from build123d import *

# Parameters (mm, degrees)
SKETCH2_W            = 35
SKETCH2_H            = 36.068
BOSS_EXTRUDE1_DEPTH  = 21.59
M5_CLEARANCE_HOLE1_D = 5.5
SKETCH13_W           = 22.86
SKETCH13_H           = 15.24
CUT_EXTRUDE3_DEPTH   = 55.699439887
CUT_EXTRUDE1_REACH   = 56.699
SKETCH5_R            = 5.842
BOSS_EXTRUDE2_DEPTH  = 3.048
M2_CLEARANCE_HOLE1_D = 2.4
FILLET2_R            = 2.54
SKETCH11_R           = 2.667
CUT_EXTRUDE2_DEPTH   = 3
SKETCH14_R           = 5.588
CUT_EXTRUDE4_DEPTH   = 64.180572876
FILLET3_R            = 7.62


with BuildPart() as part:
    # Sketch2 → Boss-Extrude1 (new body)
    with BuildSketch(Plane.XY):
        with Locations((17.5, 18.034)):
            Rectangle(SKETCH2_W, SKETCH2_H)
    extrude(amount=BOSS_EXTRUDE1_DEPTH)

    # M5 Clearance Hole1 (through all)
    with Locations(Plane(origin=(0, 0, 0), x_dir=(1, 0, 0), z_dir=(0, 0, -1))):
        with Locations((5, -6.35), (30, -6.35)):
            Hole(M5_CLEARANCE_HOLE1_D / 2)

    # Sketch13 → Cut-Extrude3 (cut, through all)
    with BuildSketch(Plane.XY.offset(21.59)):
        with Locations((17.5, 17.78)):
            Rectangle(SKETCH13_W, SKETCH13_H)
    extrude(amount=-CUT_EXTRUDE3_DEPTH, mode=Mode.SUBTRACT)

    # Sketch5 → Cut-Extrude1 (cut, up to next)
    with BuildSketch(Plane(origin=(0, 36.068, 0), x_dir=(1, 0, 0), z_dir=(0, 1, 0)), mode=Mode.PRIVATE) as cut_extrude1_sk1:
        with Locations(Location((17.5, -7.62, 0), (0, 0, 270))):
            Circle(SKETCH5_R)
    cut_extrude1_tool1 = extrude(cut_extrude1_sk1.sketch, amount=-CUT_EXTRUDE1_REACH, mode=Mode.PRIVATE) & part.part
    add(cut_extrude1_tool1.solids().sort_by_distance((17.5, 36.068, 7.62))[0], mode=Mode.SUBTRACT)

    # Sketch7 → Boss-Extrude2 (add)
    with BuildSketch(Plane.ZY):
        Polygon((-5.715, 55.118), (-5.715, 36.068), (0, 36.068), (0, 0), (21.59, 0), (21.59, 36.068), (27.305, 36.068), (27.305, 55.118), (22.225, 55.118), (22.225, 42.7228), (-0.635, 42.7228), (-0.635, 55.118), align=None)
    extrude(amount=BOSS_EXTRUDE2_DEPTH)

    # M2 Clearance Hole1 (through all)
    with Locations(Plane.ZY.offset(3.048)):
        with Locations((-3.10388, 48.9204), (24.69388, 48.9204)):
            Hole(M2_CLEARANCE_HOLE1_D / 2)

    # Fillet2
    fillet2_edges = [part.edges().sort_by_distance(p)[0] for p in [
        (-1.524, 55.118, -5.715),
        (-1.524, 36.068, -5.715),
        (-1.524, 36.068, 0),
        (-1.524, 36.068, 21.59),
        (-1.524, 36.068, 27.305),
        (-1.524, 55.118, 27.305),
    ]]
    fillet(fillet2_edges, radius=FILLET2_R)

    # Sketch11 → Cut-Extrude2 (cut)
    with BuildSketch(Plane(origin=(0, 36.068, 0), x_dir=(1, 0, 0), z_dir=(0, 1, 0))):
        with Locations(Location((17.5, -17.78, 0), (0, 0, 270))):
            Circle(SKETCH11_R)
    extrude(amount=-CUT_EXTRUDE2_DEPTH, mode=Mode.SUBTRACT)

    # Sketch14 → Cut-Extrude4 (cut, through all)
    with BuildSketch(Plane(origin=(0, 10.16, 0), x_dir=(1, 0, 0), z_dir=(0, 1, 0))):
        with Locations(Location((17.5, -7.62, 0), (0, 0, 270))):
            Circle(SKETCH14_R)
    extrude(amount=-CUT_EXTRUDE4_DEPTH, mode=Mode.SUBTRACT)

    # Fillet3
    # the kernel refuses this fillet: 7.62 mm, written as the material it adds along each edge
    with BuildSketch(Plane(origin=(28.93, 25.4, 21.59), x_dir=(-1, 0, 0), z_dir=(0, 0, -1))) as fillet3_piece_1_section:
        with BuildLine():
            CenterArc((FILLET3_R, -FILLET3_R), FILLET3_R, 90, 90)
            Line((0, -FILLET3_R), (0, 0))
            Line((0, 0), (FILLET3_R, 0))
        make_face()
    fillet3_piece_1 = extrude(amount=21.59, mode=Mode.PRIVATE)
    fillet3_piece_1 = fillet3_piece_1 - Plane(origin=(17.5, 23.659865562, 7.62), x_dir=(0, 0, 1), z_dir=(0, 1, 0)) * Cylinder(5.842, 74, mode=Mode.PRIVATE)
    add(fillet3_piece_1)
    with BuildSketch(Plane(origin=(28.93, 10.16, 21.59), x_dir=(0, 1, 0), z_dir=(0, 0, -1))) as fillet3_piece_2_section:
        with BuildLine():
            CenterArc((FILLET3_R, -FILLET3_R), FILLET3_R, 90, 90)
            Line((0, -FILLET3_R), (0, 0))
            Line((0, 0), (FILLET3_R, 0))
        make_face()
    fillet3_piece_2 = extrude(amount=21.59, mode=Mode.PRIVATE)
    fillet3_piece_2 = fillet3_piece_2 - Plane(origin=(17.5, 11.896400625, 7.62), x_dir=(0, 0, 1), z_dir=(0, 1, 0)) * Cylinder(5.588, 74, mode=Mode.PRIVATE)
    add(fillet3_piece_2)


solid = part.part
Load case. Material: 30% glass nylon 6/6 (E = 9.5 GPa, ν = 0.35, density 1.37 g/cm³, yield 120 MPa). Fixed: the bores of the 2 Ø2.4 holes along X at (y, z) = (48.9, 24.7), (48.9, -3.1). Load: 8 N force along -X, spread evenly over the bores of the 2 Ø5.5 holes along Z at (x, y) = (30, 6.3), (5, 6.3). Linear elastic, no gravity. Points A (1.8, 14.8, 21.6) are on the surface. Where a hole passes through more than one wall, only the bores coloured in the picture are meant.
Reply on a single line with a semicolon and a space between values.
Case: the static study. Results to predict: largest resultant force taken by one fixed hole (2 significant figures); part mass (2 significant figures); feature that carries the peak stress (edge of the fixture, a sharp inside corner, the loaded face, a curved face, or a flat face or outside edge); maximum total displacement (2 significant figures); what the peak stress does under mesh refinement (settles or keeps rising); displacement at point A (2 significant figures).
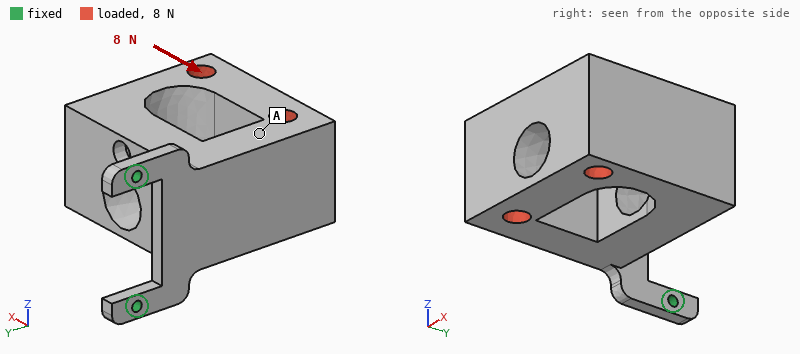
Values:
4.0 N; 28 g; edge of the fixture; 0.85 mm; keeps rising; 0.42 mm
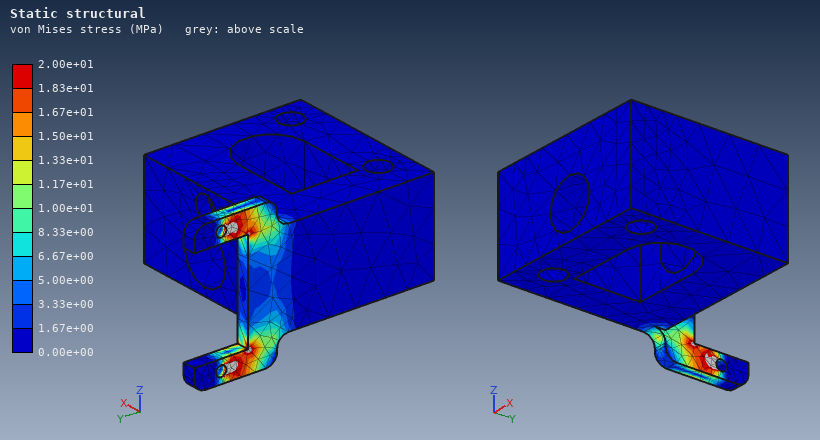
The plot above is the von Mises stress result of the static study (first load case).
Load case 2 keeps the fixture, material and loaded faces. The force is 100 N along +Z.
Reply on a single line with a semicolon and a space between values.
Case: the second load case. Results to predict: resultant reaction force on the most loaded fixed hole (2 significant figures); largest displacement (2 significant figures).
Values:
160 N; 0.52 mm
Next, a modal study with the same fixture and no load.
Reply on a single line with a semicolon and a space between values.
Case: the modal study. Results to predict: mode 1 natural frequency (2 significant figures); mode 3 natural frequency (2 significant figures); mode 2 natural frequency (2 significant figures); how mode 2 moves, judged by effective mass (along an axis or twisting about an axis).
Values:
130 Hz; 1300 Hz; 540 Hz; along Z
